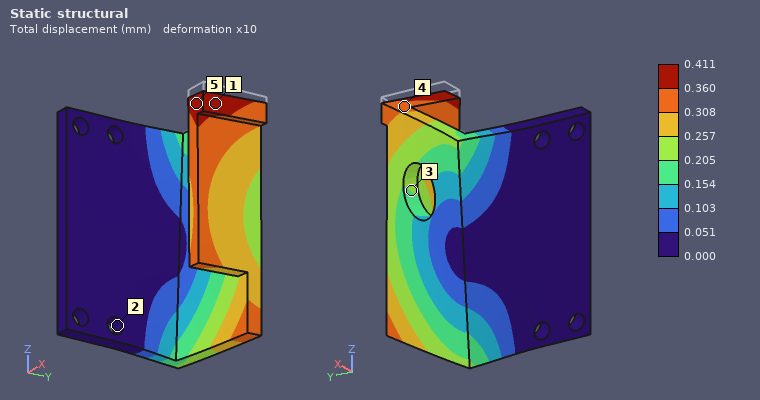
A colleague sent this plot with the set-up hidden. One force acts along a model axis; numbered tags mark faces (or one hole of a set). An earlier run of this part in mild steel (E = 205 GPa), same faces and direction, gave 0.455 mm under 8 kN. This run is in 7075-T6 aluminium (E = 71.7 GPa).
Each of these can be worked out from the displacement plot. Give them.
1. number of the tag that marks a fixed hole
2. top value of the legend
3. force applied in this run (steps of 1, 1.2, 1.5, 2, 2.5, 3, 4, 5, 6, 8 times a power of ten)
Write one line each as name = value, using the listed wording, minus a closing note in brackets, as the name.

number of the tag that marks a fixed hole = 2
top value of the legend = 0.411 mm
force applied in this run = 2.5 kN
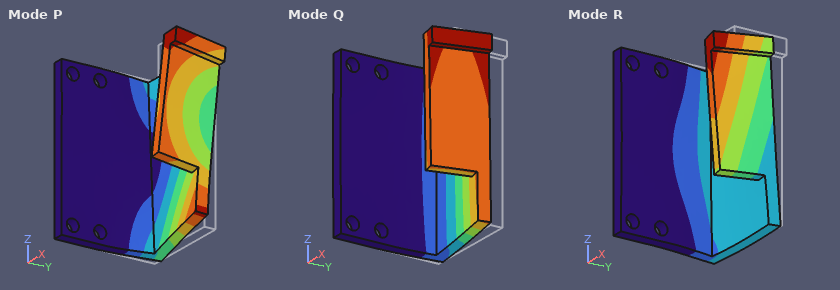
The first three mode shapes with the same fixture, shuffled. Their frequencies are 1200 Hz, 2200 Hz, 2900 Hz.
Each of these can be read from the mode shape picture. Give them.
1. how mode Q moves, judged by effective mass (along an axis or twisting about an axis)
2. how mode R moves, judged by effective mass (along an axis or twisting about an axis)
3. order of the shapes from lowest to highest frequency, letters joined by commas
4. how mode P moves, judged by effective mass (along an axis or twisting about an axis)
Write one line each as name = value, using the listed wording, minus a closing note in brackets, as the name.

how mode Q moves, judged by effective mass = along Y
how mode R moves, judged by effective mass = along X
order of the shapes from lowest to highest frequency, letters joined by commas = Q, P, R
how mode P moves, judged by effective mass = along Z
